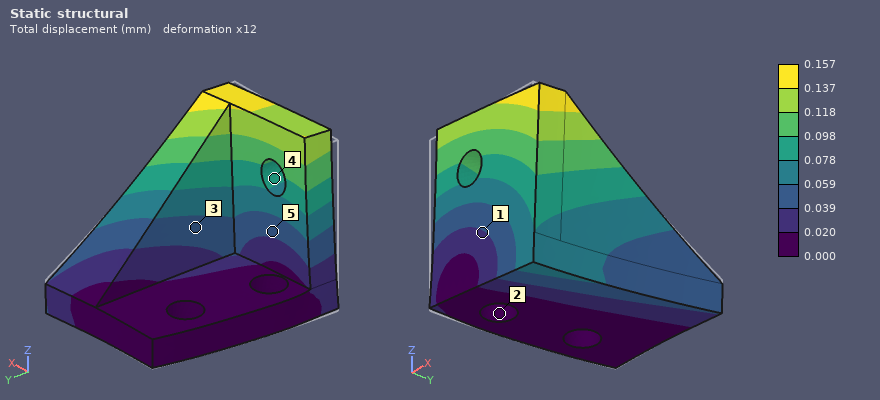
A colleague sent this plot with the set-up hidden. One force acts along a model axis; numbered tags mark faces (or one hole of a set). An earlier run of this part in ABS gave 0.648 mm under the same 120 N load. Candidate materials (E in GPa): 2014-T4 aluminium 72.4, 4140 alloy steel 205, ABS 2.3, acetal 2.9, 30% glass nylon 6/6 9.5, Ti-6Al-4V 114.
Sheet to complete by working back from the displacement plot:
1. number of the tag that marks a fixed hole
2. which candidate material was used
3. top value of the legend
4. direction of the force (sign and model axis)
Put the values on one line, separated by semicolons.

2; 30% glass nylon 6/6; 0.157 mm; +X
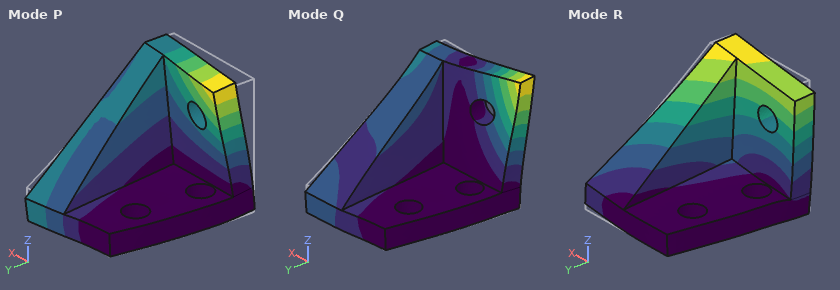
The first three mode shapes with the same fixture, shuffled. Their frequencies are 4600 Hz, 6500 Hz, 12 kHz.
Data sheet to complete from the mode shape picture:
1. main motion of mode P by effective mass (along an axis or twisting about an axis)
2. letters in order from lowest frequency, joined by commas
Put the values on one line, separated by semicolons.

along Y; R, P, Q
